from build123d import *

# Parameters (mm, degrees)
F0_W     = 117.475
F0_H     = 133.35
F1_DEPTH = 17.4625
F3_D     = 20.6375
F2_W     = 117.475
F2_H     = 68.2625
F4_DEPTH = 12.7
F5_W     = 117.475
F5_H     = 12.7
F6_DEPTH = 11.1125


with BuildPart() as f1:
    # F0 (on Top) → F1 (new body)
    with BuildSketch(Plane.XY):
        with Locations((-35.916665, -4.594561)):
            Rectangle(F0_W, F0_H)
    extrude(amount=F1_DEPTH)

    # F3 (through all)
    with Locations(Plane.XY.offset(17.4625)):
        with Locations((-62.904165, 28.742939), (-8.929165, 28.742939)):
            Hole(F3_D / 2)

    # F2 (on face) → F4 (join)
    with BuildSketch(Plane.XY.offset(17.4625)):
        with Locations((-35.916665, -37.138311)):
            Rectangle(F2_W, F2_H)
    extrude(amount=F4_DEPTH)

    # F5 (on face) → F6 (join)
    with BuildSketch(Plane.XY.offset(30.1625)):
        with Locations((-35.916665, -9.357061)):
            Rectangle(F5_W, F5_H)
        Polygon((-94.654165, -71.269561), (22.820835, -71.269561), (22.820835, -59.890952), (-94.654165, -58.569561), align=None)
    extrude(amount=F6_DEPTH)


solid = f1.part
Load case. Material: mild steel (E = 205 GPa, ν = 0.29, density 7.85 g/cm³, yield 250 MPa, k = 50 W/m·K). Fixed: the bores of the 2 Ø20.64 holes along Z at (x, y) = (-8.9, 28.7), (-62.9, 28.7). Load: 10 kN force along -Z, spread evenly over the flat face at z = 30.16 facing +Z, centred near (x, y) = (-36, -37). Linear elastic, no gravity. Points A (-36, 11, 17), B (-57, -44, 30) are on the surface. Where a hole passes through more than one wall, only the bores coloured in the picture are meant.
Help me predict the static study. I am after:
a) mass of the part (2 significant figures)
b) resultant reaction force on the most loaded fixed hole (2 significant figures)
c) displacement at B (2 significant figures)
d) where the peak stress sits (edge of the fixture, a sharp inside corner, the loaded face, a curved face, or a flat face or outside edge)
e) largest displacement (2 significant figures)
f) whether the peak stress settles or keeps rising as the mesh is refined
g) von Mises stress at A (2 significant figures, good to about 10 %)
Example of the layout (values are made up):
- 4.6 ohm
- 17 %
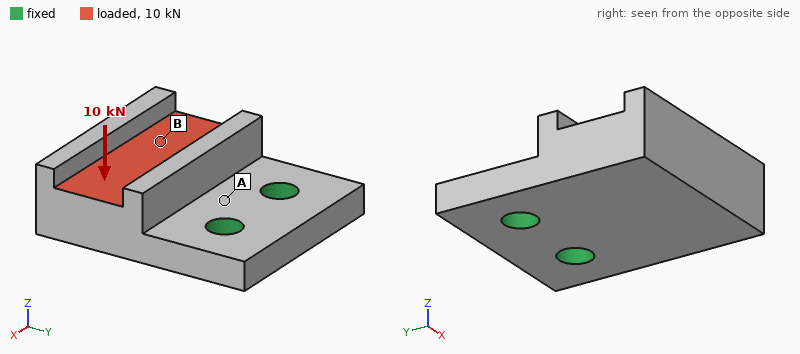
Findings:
- 3.1 kg
- 5.0 kN
- 0.084 mm
- edge of the fixture
- 0.13 mm
- keeps rising
- 61 MPa
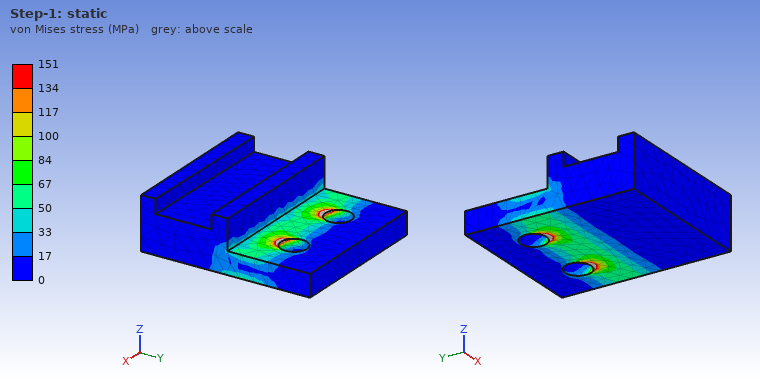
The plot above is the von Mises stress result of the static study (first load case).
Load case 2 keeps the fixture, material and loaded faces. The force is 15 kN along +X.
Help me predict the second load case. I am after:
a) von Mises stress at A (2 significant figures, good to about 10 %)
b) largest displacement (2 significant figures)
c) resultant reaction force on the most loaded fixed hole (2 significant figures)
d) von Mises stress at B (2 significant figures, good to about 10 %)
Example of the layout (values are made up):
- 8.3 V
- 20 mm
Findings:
- 29 MPa
- 27 µm
- 16 kN
- 12 MPa
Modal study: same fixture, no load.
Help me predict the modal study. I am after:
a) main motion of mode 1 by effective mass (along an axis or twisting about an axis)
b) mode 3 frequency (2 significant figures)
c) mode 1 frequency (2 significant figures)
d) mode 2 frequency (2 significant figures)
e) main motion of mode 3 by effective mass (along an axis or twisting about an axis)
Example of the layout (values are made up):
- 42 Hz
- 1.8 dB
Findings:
- along Z
- 3900 Hz
- 1200 Hz
- 3000 Hz
- along X
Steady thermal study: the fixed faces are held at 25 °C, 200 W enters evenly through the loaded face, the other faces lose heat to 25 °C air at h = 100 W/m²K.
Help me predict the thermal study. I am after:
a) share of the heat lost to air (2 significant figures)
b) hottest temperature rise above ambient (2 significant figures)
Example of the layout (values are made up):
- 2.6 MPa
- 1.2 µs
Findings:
- 57 %
- 55 K
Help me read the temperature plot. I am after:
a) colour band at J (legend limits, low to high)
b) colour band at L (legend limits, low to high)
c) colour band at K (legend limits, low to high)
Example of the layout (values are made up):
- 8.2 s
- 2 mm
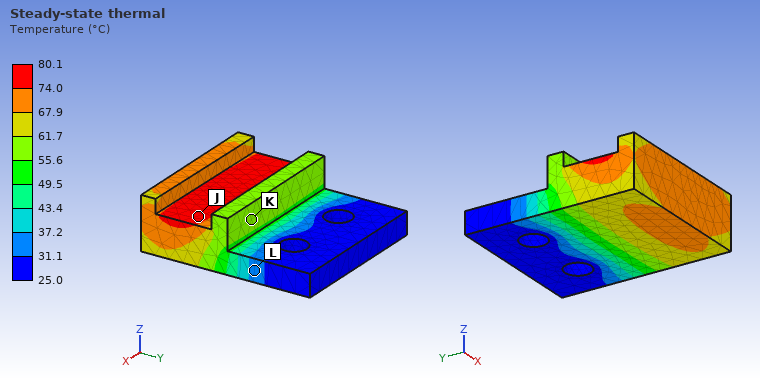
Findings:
- 74.0 to 80.1 °C
- 31.1 to 37.2 °C
- 55.6 to 61.7 °C
